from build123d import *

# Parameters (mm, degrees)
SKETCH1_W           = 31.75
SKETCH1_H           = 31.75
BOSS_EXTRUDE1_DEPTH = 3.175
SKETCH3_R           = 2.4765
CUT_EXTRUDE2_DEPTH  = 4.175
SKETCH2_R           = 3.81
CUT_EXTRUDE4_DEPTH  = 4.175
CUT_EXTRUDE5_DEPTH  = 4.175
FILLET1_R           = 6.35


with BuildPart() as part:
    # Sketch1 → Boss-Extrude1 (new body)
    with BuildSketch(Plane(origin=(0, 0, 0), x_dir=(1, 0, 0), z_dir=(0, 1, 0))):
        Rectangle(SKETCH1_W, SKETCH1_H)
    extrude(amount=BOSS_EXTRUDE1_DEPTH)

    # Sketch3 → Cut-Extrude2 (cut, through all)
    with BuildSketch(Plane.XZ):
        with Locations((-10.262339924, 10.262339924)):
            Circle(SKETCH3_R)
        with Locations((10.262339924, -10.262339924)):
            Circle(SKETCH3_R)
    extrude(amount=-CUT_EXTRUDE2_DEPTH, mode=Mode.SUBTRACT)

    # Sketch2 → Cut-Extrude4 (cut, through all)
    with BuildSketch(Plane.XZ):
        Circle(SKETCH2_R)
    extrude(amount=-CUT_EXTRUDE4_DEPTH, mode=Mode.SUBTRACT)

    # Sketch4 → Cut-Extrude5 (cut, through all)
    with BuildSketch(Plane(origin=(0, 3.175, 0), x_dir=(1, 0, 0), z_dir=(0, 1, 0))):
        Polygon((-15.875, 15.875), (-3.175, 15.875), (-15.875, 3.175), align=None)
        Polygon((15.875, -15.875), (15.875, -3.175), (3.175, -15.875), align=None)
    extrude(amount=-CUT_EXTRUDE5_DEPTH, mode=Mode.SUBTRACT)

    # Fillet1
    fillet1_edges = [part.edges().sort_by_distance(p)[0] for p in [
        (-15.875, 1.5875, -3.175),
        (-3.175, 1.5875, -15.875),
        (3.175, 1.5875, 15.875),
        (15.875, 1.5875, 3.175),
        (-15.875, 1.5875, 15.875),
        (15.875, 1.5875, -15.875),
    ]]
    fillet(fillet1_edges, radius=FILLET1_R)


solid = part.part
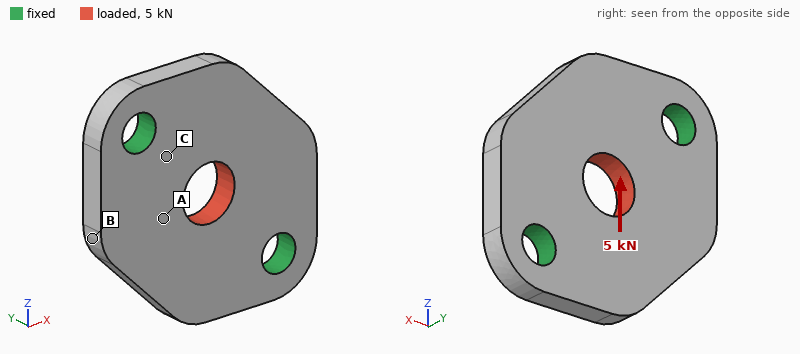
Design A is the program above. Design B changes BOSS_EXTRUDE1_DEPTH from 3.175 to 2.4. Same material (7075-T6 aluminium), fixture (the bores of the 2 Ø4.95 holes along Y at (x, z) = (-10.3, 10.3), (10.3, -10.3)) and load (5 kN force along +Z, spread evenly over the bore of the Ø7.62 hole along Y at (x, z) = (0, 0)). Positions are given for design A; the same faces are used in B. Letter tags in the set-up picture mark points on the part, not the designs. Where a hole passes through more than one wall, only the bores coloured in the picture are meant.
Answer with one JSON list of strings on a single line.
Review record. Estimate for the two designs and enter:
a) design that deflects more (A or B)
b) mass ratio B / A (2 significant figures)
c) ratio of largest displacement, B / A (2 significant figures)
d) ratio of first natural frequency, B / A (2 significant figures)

["B", "0.76", "1.3", "0.79"]
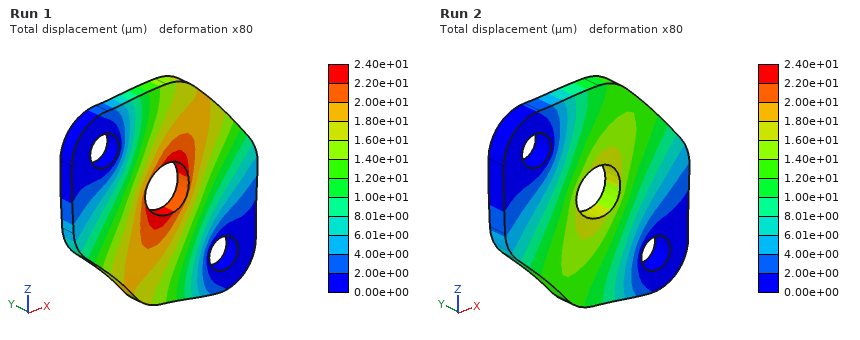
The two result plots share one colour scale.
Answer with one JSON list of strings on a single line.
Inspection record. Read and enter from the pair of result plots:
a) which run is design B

["Run 1"]
